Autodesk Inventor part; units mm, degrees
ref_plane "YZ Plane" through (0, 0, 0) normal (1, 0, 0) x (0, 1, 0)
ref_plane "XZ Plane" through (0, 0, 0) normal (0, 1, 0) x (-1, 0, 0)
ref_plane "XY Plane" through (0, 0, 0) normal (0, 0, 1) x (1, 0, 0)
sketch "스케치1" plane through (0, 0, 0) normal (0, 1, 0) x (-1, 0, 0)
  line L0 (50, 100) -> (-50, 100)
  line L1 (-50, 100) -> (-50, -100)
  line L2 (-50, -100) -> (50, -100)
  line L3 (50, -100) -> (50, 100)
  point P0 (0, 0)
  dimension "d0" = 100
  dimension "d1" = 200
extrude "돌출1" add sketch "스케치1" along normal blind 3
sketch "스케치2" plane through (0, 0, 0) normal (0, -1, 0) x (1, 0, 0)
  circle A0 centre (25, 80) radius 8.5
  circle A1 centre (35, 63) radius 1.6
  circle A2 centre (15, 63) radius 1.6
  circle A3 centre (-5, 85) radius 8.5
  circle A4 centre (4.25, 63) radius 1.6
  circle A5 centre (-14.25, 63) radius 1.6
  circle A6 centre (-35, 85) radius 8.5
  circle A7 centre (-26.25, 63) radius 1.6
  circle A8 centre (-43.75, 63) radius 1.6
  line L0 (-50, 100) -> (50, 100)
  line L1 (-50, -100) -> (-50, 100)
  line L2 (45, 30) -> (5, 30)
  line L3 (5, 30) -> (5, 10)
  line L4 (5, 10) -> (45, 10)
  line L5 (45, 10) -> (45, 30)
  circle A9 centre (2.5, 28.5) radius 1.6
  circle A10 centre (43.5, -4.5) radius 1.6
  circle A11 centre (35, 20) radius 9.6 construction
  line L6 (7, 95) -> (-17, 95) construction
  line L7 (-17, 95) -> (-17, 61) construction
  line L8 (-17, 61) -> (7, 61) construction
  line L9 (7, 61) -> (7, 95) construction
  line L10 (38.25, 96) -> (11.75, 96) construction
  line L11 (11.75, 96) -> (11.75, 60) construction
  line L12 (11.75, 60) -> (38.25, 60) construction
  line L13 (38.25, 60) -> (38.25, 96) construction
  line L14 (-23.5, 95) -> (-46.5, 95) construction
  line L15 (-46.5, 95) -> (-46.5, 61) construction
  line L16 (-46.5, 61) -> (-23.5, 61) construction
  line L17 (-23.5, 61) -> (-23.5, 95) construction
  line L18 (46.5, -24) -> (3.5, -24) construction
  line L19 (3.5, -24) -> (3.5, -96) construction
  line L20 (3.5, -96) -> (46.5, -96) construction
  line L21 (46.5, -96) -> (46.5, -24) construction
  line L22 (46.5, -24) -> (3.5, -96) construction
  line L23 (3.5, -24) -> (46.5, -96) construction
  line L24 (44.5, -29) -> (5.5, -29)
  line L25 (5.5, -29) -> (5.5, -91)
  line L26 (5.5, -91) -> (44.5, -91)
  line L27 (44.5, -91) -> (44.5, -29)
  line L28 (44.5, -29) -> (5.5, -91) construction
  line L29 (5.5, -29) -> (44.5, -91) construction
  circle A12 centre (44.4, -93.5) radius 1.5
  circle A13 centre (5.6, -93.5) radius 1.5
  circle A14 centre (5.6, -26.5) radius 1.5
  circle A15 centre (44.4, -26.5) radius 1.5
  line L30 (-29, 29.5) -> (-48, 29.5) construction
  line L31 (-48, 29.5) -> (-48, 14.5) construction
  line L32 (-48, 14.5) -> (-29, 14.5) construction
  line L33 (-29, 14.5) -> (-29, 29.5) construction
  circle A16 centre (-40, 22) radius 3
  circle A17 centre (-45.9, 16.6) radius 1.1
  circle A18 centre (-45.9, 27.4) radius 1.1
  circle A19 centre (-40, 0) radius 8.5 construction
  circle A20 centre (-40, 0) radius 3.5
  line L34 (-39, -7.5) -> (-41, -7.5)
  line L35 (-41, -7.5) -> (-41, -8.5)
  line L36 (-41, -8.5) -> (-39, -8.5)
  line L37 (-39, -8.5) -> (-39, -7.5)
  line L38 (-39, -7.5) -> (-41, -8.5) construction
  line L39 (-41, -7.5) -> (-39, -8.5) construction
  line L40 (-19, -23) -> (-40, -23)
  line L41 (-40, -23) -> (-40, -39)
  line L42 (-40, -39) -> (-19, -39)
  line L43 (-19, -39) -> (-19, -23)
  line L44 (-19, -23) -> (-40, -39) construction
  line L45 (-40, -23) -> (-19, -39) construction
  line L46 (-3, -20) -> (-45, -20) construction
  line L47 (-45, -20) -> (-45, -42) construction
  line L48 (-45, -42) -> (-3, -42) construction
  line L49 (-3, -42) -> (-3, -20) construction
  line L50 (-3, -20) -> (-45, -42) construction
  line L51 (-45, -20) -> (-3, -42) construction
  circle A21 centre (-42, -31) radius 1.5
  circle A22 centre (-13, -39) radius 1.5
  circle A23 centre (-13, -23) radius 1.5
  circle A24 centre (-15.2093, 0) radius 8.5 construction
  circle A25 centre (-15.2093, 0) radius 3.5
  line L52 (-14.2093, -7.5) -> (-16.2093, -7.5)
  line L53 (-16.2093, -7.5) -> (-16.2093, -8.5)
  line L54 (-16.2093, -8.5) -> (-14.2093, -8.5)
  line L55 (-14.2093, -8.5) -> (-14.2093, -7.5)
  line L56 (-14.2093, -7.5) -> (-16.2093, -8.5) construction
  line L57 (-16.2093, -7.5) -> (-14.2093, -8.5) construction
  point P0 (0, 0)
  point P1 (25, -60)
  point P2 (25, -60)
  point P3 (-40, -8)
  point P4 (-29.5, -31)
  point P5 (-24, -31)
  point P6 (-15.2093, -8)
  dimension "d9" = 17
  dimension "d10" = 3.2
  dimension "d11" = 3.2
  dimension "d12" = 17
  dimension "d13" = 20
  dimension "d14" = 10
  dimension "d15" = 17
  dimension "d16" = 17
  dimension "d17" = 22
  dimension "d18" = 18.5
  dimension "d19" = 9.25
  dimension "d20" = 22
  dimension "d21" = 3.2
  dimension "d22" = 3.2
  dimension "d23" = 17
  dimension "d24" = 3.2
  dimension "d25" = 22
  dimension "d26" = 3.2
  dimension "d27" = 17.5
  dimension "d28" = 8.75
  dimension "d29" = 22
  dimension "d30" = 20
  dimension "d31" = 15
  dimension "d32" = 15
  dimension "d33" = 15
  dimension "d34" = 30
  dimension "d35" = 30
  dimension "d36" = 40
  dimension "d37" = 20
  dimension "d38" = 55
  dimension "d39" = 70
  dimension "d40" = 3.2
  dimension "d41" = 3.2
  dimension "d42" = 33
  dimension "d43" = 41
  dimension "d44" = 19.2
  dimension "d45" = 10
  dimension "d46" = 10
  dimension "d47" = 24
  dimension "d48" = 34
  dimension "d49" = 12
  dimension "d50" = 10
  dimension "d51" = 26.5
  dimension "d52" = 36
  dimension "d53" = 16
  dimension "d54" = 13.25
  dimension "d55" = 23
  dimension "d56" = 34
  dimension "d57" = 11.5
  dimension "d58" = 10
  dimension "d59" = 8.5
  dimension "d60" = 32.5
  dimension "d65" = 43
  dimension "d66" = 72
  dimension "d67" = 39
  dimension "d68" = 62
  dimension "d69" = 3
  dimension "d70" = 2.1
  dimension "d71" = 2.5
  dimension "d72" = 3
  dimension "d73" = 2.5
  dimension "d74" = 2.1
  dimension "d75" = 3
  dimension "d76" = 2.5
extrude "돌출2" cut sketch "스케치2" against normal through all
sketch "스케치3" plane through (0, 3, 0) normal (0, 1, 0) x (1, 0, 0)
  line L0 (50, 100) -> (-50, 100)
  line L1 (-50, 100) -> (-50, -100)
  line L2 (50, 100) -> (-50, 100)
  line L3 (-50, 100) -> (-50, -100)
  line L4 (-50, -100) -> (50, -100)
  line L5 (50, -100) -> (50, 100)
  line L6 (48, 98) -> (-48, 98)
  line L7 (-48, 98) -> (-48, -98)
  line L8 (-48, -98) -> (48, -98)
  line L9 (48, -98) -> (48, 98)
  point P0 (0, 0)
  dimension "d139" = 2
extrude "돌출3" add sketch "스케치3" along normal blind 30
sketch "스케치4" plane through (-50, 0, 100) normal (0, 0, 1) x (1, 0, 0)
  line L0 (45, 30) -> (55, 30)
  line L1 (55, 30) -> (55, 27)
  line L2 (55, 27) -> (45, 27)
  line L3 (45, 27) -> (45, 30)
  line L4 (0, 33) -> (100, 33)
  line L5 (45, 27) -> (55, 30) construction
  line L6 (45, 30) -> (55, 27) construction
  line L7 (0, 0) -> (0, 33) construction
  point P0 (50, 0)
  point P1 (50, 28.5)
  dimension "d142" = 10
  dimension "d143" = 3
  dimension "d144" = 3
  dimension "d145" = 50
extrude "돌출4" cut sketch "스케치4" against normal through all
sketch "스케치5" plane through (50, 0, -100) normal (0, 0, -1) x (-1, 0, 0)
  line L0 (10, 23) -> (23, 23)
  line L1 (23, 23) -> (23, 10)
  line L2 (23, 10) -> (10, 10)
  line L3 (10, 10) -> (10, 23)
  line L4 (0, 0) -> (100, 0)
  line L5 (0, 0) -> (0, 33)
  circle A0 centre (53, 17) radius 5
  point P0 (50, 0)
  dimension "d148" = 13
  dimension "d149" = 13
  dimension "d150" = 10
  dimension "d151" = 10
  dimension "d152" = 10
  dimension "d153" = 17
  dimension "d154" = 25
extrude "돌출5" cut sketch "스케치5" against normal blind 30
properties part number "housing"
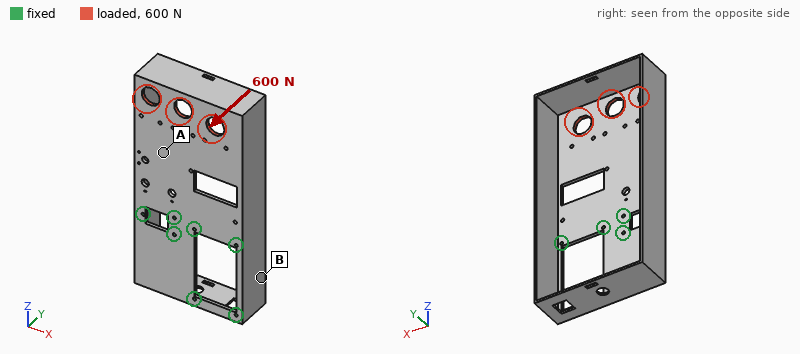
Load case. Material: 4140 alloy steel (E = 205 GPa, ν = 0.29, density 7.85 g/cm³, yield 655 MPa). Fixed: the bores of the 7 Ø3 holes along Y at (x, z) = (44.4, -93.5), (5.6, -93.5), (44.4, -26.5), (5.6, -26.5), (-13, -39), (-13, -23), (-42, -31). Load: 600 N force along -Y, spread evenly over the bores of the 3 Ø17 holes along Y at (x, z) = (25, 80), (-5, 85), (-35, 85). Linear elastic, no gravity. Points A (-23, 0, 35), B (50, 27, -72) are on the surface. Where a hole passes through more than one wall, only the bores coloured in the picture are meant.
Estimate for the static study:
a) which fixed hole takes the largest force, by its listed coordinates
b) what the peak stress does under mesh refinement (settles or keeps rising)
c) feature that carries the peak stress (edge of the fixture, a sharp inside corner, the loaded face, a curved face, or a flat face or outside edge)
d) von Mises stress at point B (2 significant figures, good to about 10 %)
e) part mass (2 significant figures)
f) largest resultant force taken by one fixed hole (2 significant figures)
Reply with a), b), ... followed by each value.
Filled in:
a) (5.6, -93.5)
b) keeps rising
c) edge of the fixture
d) 14 MPa
e) 640 g
f) 1.2 kN
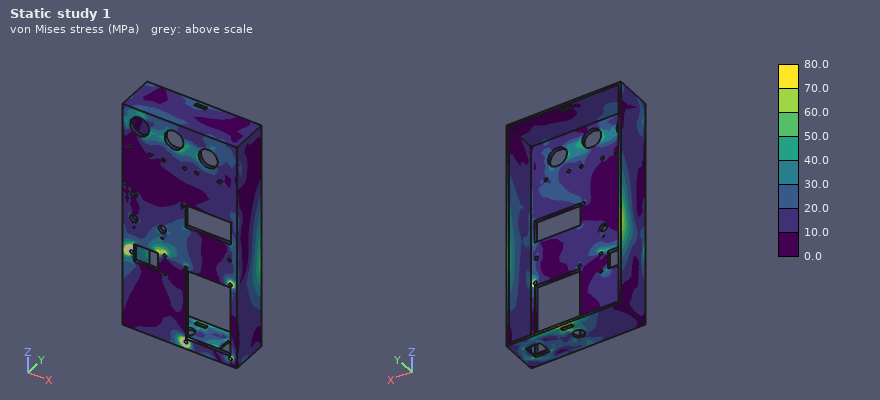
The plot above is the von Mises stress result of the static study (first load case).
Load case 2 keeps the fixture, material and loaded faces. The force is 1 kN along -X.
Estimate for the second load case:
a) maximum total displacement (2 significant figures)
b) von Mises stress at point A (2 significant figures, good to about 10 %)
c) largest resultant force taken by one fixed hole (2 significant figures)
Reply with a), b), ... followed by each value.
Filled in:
a) 55 µm
b) 7.7 MPa
c) 1.1 kN
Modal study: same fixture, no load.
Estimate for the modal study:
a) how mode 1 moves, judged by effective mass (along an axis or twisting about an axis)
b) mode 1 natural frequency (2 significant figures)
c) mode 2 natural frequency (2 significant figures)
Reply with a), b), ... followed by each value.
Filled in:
a) along Y
b) 570 Hz
c) 860 Hz
